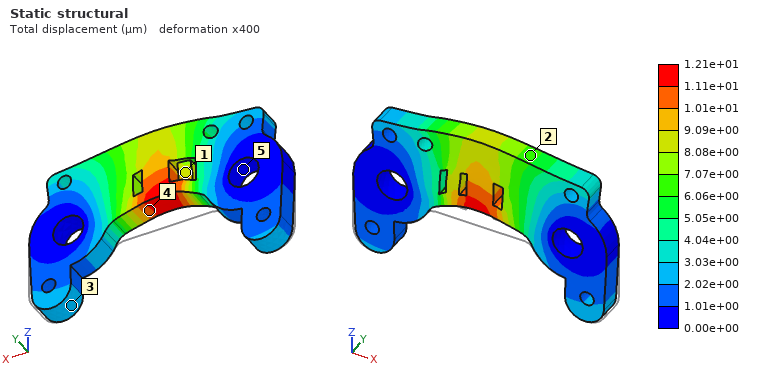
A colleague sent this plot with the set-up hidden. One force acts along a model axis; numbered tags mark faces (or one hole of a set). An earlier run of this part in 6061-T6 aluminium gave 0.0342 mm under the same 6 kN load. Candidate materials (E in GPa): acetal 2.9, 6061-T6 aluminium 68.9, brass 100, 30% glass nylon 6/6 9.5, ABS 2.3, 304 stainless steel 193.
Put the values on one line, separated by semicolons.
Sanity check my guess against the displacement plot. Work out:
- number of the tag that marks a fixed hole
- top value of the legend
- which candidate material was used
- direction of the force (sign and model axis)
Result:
5; 1.21e+01 µm; 304 stainless steel; +Z
